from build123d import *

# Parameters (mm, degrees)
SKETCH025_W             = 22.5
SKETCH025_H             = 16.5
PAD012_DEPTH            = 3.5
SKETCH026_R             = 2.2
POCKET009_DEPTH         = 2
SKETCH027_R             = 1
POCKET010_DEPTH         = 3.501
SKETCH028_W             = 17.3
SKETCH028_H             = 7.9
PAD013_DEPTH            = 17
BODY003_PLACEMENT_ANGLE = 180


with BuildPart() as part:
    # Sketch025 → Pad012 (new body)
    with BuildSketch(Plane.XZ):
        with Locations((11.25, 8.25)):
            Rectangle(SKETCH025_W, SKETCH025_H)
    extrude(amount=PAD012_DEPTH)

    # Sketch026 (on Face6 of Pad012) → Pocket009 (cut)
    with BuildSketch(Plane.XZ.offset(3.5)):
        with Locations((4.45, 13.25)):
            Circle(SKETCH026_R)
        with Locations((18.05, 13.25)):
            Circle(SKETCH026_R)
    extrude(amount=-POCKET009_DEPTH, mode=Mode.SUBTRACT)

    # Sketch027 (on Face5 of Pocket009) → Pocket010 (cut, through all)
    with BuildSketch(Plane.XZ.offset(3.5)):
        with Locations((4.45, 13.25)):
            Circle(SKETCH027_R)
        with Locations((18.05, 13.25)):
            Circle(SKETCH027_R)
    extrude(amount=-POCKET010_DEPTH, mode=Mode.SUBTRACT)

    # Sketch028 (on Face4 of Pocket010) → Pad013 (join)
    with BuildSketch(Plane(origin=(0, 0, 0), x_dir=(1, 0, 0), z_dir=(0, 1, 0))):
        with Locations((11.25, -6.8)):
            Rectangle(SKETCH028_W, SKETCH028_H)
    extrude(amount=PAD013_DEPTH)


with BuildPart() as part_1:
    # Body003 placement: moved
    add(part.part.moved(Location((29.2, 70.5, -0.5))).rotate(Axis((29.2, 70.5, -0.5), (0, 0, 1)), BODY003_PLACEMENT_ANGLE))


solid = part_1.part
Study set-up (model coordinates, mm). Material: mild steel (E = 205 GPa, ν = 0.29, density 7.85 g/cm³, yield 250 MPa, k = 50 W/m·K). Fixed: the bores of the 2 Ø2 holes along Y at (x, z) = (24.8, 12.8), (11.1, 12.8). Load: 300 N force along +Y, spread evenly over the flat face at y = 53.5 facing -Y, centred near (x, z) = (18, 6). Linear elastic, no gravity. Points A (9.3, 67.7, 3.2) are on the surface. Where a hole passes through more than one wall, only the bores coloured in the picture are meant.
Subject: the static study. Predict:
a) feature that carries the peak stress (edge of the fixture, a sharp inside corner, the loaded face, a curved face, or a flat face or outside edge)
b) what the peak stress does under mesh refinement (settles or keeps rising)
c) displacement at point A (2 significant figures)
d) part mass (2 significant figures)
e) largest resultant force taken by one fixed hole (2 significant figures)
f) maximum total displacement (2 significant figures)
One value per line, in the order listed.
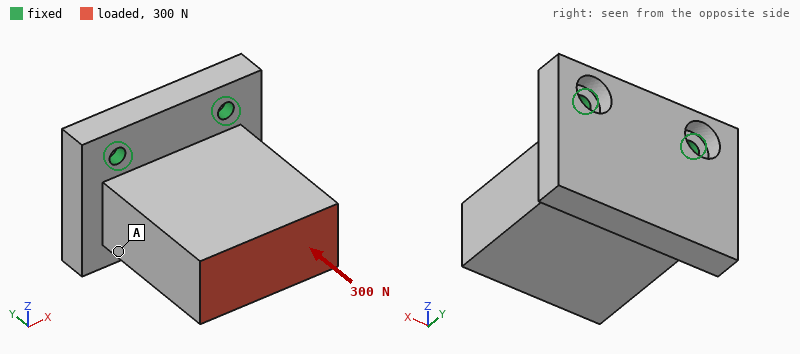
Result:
edge of the fixture
keeps rising
15 µm
28 g
150 N
31 µm
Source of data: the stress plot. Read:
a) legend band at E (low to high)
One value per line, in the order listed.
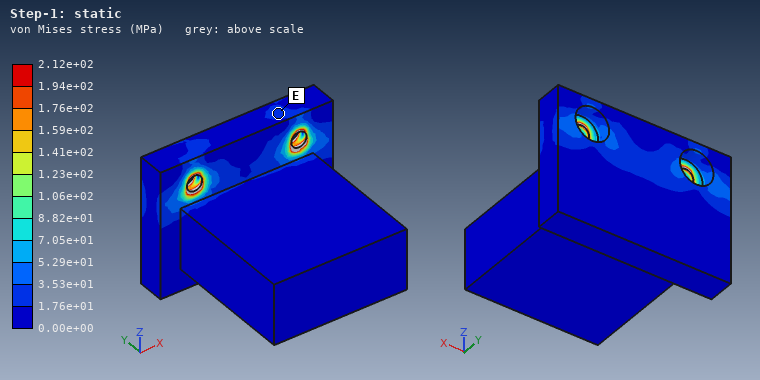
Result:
1.76e+01 to 3.53e+01 MPa
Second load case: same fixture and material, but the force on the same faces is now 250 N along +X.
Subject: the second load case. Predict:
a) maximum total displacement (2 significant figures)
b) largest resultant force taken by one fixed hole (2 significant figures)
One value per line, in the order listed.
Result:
8.1 µm
350 N
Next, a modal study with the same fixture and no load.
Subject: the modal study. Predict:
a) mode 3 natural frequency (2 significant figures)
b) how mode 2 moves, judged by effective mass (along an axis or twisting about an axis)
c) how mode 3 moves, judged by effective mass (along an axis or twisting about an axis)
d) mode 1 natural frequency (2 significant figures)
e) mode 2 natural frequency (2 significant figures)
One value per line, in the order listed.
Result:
18 kHz
along X
along Y
2900 Hz
10 kHz
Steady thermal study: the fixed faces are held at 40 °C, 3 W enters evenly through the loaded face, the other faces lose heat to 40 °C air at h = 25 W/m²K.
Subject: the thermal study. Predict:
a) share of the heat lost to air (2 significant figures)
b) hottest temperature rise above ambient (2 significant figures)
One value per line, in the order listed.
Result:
11 %
14 K
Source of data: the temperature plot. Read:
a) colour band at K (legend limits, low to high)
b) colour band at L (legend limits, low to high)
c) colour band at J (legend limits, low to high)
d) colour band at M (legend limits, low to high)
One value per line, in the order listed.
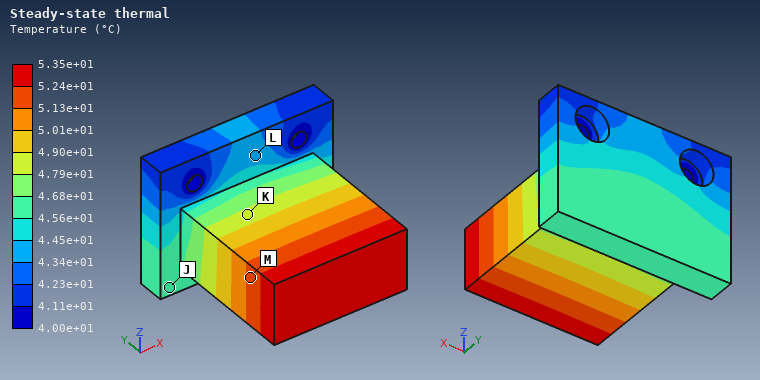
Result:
4.79e+01 to 4.90e+01 °C
4.34e+01 to 4.45e+01 °C
4.56e+01 to 4.68e+01 °C
5.13e+01 to 5.24e+01 °C
